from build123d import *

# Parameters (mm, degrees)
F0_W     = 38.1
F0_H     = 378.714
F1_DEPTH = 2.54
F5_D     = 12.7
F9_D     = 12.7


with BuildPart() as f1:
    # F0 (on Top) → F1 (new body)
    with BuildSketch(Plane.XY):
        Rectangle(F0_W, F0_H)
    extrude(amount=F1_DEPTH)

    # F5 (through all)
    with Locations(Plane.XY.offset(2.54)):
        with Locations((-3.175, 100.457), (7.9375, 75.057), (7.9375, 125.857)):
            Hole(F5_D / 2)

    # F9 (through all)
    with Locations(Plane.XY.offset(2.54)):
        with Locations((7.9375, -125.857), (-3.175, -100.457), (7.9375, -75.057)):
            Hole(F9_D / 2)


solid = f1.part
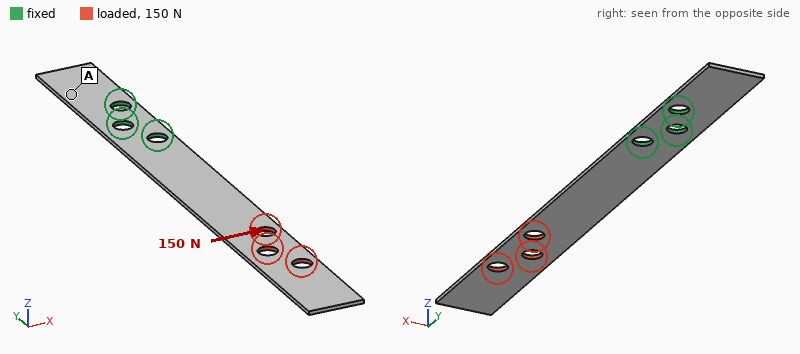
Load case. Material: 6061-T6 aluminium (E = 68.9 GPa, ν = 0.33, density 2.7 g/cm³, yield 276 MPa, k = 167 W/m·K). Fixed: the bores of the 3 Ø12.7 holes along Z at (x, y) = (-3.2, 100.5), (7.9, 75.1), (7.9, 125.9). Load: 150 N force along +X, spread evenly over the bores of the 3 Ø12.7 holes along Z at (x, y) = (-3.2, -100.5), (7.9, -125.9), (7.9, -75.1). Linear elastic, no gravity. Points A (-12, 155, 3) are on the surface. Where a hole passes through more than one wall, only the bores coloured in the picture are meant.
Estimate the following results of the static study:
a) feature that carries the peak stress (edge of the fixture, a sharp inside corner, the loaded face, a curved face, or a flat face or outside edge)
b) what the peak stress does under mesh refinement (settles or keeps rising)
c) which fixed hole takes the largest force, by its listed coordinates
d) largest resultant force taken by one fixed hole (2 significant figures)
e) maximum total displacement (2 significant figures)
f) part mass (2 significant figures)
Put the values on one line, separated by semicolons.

edge of the fixture; keeps rising; (7.9, 75.1); 760 N; 0.67 mm; 94 g
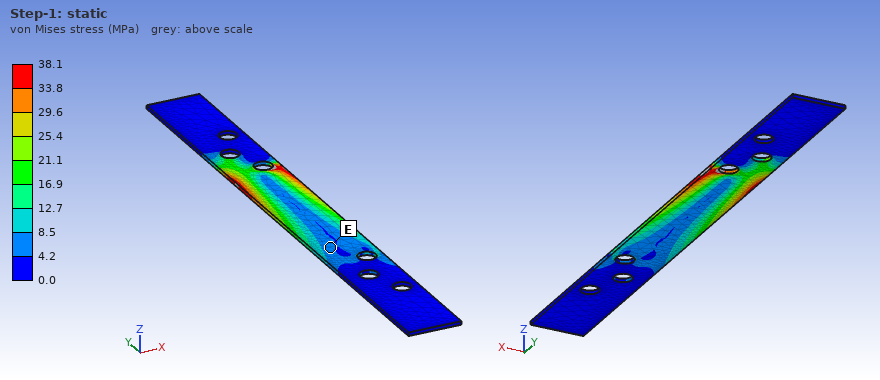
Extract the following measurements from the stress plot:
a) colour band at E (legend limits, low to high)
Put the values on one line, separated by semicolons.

4.2 to 8.5 MPa
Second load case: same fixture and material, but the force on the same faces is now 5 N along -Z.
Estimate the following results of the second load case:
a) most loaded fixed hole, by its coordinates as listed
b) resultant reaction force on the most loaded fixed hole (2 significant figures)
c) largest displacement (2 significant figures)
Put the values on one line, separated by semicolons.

(7.9, 75.1); 13 N; 4.2 mm
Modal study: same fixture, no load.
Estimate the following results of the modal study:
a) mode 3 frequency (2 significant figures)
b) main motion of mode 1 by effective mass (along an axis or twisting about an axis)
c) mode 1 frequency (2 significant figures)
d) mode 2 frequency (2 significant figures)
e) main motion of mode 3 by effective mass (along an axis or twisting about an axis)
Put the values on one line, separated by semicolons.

390 Hz; along Z; 31 Hz; 190 Hz; twisting about Y
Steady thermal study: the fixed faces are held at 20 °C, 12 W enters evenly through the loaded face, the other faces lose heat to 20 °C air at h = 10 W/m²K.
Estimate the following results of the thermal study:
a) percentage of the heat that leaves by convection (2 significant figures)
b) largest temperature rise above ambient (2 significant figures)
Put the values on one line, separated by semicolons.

63 %; 60 K
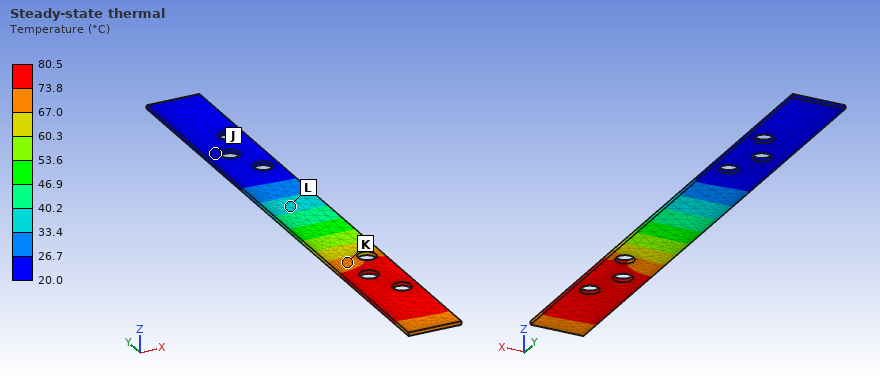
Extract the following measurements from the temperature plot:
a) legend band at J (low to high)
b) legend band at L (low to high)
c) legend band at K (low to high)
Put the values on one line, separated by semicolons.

20.0 to 26.7 °C; 33.4 to 40.2 °C; 67.0 to 73.8 °C
